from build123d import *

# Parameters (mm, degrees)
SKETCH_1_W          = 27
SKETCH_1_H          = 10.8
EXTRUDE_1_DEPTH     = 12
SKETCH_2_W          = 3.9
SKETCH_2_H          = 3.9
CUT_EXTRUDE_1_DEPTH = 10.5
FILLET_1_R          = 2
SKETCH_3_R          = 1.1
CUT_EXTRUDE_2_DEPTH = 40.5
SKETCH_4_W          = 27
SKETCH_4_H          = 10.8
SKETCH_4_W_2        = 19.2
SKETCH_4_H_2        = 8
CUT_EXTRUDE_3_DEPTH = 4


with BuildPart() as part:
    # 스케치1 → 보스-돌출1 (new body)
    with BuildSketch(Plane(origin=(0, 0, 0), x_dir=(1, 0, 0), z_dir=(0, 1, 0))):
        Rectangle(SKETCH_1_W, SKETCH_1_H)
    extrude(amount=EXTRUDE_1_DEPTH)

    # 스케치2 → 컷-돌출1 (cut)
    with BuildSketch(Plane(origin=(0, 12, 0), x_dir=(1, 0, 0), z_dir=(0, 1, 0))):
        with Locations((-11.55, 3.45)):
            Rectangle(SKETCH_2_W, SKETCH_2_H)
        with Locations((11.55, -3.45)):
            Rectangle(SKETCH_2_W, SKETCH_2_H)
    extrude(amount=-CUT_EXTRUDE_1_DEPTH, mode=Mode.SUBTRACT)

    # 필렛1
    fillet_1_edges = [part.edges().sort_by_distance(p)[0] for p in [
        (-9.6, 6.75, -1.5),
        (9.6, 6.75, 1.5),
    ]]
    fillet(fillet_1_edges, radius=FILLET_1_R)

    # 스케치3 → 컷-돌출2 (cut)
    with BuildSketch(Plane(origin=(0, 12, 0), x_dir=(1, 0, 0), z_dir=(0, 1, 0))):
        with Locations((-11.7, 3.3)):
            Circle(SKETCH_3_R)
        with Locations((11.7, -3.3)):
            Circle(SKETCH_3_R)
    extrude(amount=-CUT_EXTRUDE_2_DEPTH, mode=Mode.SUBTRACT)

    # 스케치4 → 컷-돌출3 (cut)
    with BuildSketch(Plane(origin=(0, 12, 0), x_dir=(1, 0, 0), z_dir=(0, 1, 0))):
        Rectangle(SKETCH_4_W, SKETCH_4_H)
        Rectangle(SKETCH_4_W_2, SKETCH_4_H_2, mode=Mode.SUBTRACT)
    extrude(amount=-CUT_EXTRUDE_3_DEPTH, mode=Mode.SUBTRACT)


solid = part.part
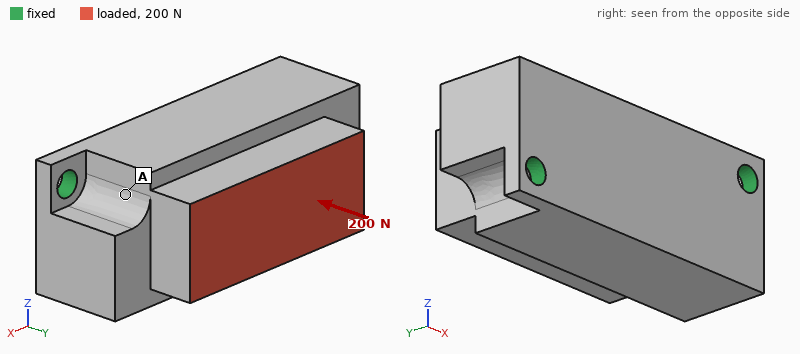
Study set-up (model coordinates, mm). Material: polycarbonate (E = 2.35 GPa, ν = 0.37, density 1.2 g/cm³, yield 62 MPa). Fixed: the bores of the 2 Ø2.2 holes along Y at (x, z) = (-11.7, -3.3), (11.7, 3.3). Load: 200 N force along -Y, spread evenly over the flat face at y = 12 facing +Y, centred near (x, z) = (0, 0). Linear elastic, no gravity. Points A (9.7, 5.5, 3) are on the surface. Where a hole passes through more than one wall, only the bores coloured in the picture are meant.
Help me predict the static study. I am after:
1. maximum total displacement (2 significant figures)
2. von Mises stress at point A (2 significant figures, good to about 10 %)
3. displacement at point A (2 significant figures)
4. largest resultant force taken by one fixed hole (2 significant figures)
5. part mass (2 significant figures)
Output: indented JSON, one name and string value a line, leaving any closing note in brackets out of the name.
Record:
{
  "maximum total displacement": "54 µm",
  "von Mises stress at point A": "4.0 MPa",
  "displacement at point A": "40 µm",
  "largest resultant force taken by one fixed hole": "110 N",
  "part mass": "3.3 g"
}
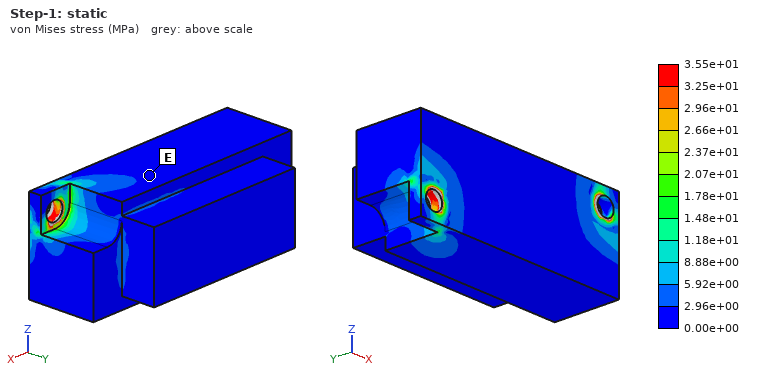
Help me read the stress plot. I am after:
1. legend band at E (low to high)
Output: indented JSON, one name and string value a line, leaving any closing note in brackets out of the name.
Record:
{
  "legend band at E": "0.00e+00 to 2.96e+00 MPa"
}
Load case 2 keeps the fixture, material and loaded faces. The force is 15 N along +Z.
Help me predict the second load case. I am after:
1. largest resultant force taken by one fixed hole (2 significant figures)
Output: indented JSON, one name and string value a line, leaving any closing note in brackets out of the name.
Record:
{
  "largest resultant force taken by one fixed hole": "8.4 N"
}
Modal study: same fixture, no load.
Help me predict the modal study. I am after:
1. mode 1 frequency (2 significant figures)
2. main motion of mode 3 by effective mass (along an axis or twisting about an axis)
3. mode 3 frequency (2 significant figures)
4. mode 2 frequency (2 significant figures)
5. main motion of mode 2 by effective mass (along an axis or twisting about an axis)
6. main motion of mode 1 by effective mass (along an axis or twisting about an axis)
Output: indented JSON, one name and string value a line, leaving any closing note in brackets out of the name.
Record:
{
  "mode 1 frequency": "1400 Hz",
  "main motion of mode 3 by effective mass": "along X",
  "mode 3 frequency": "7300 Hz",
  "mode 2 frequency": "5700 Hz",
  "main motion of mode 2 by effective mass": "along Y",
  "main motion of mode 1 by effective mass": "along Z"
}
